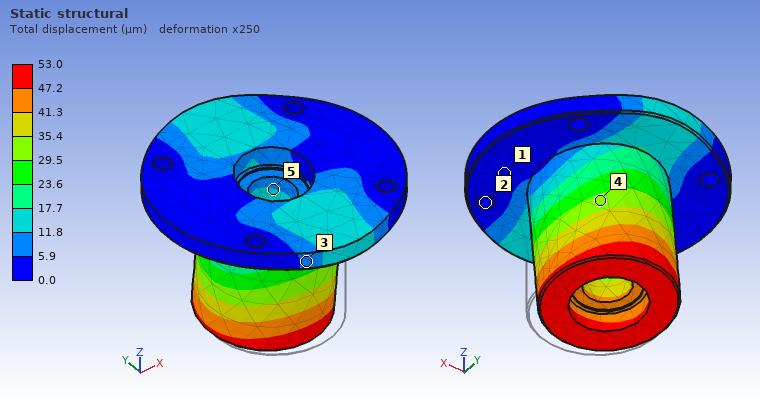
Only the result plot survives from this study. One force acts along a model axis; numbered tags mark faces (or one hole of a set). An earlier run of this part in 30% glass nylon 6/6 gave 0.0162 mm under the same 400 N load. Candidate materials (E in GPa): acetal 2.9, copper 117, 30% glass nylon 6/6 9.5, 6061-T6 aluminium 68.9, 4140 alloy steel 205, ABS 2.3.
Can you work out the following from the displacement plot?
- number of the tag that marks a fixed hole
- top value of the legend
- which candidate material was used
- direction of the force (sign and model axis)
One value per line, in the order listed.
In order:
2
53.0 µm
acetal
+Y
